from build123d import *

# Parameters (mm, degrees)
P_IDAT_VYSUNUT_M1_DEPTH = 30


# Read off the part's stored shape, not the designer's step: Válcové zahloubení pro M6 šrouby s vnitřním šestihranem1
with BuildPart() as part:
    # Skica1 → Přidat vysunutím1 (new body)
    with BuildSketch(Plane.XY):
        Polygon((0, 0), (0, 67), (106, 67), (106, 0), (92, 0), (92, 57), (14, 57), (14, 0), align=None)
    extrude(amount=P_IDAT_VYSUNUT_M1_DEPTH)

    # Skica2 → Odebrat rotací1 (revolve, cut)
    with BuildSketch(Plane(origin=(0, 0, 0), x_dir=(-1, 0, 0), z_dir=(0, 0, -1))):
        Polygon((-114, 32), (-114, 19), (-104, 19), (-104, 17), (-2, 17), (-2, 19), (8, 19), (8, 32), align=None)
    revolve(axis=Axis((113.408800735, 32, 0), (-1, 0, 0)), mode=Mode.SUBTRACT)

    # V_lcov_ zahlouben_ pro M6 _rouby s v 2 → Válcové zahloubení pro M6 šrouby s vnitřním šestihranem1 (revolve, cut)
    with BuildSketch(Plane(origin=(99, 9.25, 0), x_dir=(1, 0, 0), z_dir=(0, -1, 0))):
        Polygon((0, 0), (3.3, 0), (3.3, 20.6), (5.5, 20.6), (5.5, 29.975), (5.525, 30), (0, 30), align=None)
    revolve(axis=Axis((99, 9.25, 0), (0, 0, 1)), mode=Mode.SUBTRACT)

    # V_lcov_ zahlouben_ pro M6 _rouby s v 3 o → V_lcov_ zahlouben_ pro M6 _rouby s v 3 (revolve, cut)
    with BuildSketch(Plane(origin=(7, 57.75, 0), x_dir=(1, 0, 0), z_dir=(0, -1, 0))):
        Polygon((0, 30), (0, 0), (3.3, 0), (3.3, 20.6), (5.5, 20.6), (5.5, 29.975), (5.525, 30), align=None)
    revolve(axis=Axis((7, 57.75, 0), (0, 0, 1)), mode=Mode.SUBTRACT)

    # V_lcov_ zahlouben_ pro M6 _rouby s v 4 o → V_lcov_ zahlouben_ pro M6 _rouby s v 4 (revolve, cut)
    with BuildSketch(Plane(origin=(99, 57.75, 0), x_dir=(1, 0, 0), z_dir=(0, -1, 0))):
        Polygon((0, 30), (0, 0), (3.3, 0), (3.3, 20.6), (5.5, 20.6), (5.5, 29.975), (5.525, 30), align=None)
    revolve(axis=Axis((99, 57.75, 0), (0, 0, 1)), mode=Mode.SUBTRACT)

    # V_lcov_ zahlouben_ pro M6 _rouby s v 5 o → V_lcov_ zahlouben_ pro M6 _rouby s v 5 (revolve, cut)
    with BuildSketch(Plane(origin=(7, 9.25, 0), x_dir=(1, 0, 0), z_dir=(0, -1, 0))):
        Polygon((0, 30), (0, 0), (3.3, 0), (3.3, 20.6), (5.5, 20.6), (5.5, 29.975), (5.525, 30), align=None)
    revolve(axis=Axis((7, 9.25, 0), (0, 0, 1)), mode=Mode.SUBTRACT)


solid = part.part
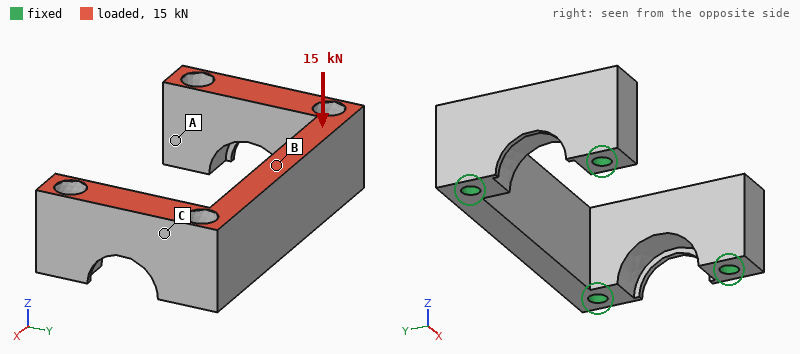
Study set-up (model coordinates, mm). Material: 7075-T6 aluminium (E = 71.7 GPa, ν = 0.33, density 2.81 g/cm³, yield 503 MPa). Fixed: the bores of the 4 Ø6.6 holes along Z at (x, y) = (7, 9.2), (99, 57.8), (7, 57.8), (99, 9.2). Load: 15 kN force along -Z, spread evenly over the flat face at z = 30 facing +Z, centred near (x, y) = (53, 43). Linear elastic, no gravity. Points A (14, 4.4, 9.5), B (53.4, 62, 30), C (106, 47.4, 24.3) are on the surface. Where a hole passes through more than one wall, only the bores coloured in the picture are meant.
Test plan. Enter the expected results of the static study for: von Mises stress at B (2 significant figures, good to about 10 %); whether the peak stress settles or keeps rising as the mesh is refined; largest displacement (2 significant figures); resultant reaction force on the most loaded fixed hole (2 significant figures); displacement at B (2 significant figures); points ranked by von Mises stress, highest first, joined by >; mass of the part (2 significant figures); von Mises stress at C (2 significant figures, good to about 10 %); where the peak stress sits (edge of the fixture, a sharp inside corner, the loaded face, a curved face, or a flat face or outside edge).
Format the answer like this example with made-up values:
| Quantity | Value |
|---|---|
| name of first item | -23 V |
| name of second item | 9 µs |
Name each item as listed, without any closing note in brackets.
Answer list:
| Quantity | Value |
|---|---|
| von Mises stress at B | 22 MPa |
| whether the peak stress settles or keeps rising as the mesh is refined | keeps rising |
| largest displacement | 21 µm |
| resultant reaction force on the most loaded fixed hole | 5.3 kN |
| displacement at B | 21 µm |
| points ranked by von Mises stress, highest first, joined by > | B > C > A |
| mass of the part | 180 g |
| von Mises stress at C | 9.7 MPa |
| where the peak stress sits | edge of the fixture |
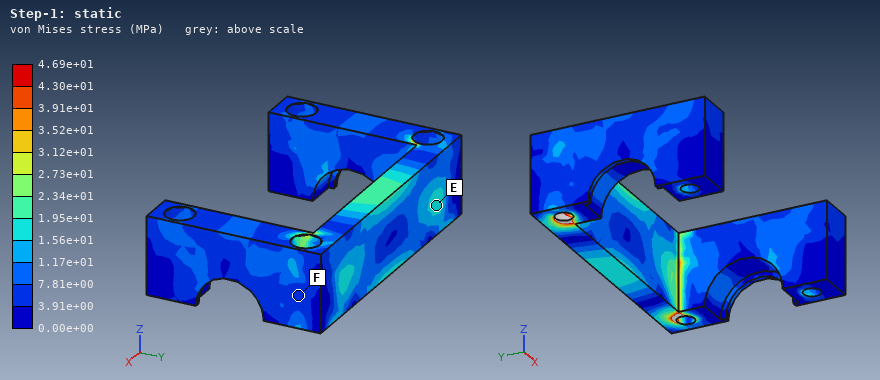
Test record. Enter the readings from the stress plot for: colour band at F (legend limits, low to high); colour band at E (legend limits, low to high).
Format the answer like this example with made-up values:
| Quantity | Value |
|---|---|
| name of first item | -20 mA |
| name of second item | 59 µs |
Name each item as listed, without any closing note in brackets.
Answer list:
| Quantity | Value |
|---|---|
| colour band at F | 3.91e+00 to 7.81e+00 MPa |
| colour band at E | 1.56e+01 to 1.95e+01 MPa |
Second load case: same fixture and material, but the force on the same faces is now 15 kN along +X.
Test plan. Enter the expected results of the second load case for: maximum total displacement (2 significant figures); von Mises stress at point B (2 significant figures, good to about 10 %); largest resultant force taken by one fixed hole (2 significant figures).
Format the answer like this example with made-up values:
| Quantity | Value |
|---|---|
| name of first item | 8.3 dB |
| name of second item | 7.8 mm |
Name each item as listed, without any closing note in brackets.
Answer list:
| Quantity | Value |
|---|---|
| maximum total displacement | 34 µm |
| von Mises stress at point B | 11 MPa |
| largest resultant force taken by one fixed hole | 5.3 kN |
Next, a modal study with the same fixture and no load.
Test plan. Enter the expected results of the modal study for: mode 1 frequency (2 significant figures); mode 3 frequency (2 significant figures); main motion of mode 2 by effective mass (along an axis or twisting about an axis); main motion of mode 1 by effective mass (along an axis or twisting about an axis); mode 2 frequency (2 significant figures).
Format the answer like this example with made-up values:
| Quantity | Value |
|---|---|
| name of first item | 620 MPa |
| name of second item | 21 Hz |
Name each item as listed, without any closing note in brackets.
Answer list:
| Quantity | Value |
|---|---|
| mode 1 frequency | 6000 Hz |
| mode 3 frequency | 11 kHz |
| main motion of mode 2 by effective mass | along Z |
| main motion of mode 1 by effective mass | along Y |
| mode 2 frequency | 11 kHz |
